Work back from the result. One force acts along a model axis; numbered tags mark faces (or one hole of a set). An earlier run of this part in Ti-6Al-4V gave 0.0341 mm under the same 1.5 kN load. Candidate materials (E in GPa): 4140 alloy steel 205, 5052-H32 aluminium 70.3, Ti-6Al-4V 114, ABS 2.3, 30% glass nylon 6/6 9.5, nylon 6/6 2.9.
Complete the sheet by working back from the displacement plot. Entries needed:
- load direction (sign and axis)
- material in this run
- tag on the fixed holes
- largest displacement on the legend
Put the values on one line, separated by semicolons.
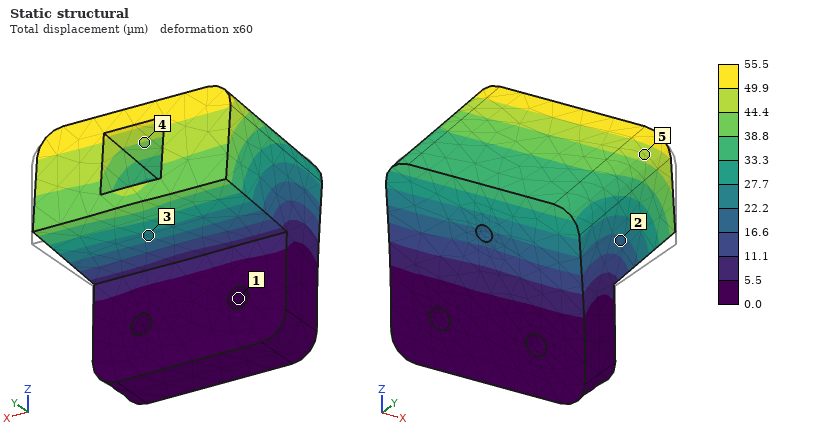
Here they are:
+Z; 5052-H32 aluminium; 1; 55.5 µm
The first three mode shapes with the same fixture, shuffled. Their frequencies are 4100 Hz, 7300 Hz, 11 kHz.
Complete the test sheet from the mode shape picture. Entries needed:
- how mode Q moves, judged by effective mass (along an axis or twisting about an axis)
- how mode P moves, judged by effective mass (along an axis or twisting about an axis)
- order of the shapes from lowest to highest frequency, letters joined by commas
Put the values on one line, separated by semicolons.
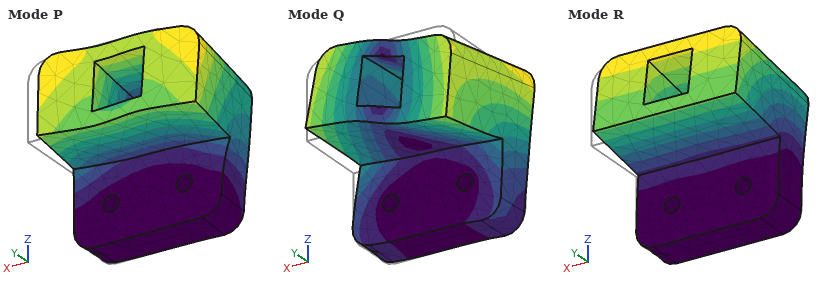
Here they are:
along X; along X; R, P, Q
